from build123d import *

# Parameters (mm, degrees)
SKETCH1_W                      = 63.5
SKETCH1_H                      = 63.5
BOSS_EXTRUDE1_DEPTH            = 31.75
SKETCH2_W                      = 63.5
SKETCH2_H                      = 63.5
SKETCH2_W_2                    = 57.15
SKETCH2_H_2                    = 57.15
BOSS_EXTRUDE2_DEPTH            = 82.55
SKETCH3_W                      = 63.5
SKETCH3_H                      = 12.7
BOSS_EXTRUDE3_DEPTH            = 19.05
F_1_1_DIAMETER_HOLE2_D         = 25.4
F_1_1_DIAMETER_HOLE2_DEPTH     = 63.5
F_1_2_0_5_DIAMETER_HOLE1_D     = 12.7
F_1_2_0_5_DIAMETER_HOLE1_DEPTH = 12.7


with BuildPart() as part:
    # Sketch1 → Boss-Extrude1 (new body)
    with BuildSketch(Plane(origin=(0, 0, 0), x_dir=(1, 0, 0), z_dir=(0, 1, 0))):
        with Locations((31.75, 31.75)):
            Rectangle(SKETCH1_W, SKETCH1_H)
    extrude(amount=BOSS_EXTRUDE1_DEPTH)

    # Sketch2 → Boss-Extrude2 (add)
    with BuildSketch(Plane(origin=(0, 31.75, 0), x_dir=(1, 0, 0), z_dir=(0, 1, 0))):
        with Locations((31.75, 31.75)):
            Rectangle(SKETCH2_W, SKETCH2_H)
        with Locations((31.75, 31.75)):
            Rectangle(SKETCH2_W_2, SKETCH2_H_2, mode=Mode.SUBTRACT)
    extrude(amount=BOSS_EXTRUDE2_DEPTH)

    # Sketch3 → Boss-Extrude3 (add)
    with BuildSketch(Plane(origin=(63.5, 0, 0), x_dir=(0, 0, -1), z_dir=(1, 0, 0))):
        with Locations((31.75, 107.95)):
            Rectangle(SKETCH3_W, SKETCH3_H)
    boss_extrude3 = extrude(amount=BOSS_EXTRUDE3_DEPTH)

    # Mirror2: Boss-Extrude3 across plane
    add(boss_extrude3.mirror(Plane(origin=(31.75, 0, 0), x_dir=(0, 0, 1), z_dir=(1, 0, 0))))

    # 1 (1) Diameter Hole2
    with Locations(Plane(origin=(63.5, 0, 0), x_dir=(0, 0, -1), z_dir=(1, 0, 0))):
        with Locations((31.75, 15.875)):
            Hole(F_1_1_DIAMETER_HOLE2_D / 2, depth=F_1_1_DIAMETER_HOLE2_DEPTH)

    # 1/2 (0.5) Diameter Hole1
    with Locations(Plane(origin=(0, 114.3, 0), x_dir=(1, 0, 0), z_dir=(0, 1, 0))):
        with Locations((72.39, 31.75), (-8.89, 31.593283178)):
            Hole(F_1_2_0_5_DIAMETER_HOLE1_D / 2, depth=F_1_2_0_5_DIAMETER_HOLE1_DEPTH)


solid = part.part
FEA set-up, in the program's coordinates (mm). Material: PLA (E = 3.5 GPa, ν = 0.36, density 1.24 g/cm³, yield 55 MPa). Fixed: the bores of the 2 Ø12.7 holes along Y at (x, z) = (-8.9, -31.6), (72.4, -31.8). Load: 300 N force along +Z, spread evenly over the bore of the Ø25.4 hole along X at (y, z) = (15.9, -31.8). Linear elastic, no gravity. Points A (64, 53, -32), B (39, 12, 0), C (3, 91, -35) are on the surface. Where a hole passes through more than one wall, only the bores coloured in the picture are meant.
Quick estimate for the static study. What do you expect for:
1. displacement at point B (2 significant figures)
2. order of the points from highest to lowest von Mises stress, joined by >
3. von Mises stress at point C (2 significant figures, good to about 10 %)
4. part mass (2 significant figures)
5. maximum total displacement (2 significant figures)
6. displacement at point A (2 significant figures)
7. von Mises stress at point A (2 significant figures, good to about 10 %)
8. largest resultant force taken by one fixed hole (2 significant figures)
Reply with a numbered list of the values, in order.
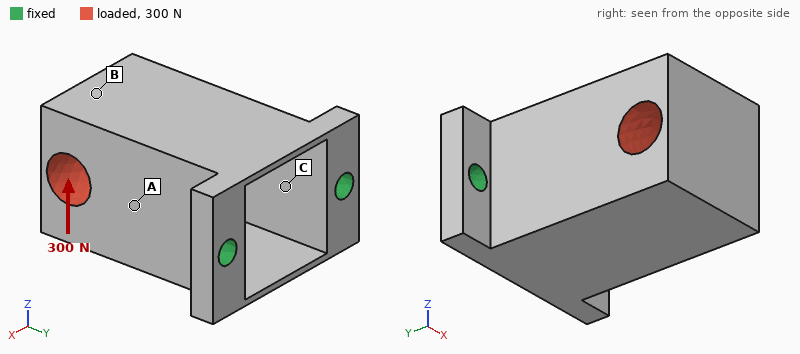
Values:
1. 0.52 mm
2. C > A > B
3. 3.2 MPa
4. 230 g
5. 0.57 mm
6. 0.27 mm
7. 1.7 MPa
8. 150 N
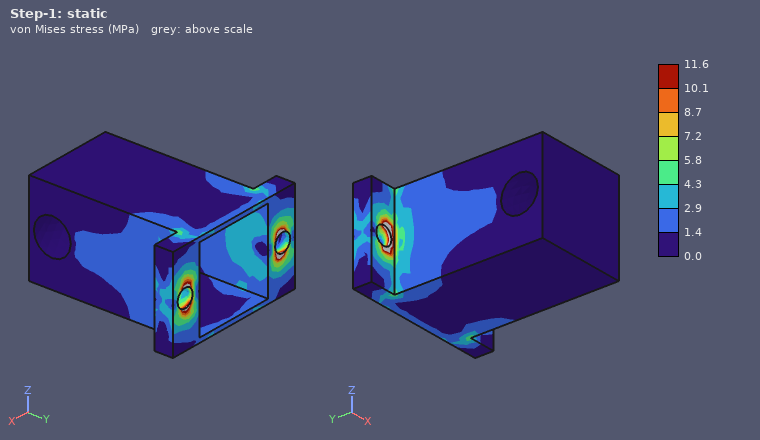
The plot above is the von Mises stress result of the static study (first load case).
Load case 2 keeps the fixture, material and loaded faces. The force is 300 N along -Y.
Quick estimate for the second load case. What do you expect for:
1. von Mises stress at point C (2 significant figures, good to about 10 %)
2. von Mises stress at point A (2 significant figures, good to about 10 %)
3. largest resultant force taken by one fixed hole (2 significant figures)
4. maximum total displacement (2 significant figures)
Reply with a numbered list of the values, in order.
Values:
1. 0.87 MPa
2. 0.52 MPa
3. 150 N
4. 22 µm
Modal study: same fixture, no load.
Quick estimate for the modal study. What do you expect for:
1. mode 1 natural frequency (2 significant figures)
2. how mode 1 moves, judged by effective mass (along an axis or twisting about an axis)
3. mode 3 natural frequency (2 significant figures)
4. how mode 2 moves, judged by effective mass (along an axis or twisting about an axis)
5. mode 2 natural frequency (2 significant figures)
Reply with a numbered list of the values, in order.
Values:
1. 330 Hz
2. along Z
3. 1400 Hz
4. along X
5. 570 Hz
